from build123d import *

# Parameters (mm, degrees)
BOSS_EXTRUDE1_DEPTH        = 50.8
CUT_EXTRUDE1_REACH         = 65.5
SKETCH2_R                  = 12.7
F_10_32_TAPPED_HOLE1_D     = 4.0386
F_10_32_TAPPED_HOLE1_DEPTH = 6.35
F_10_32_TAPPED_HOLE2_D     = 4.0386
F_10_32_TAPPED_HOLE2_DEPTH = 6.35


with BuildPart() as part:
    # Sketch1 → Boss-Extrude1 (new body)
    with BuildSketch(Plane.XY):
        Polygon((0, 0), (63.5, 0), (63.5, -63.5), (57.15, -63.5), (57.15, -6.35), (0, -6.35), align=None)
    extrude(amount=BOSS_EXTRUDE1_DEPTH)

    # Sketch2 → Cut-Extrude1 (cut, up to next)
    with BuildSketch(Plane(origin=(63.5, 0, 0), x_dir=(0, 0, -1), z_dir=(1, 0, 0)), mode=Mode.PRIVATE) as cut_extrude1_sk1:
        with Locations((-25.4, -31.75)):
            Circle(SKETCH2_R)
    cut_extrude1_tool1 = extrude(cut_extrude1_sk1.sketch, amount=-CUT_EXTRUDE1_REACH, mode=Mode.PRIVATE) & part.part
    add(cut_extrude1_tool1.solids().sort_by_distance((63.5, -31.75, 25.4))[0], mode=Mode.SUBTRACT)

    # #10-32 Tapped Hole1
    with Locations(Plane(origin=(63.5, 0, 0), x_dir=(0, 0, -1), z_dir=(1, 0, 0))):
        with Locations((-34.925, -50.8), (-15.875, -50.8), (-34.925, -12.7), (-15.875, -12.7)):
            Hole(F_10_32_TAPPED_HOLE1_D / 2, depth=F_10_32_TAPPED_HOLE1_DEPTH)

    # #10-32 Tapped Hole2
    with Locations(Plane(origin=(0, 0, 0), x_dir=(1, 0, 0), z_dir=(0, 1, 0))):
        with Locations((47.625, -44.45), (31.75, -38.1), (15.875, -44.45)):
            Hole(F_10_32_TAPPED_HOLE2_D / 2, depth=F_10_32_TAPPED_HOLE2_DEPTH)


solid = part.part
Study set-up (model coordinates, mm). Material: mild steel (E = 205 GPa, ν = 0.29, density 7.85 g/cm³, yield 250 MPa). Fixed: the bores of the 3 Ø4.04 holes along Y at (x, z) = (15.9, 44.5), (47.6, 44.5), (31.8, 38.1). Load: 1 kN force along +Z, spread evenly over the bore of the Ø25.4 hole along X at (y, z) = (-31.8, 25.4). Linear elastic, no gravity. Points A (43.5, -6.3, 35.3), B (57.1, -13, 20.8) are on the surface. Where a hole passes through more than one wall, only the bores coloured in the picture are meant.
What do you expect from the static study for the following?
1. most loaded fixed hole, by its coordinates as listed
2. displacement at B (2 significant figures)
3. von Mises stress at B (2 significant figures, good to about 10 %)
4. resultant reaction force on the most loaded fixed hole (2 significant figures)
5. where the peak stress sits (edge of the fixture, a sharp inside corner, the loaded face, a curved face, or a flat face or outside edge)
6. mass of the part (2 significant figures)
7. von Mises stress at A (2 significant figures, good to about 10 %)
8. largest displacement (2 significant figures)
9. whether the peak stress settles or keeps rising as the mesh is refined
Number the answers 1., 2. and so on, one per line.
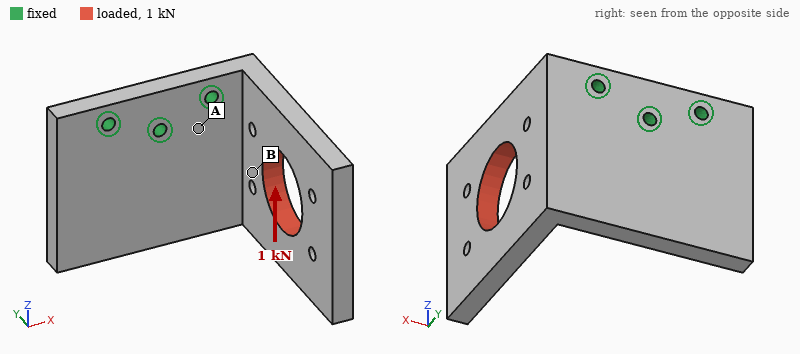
1. (47.6, 44.5)
2. 0.038 mm
3. 18 MPa
4. 1.3 kN
5. edge of the fixture
6. 280 g
7. 56 MPa
8. 0.13 mm
9. keeps rising
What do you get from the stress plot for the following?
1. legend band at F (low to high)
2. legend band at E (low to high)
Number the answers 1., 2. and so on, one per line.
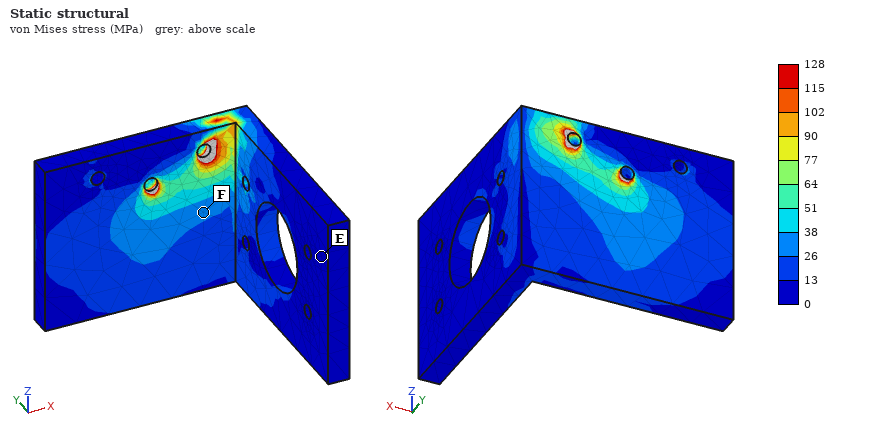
1. 26 to 38 MPa
2. 0 to 13 MPa
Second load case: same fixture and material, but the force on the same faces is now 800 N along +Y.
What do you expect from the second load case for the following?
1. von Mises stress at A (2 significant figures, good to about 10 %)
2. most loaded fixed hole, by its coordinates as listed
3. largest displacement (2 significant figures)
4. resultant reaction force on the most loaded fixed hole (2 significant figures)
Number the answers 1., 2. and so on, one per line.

1. 36 MPa
2. (47.6, 44.5)
3. 82 µm
4. 740 N
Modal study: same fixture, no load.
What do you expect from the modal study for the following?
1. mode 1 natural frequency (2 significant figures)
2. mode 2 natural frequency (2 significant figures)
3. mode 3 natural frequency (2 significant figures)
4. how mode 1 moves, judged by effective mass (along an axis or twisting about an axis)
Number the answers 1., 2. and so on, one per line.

1. 930 Hz
2. 1400 Hz
3. 3000 Hz
4. along X
